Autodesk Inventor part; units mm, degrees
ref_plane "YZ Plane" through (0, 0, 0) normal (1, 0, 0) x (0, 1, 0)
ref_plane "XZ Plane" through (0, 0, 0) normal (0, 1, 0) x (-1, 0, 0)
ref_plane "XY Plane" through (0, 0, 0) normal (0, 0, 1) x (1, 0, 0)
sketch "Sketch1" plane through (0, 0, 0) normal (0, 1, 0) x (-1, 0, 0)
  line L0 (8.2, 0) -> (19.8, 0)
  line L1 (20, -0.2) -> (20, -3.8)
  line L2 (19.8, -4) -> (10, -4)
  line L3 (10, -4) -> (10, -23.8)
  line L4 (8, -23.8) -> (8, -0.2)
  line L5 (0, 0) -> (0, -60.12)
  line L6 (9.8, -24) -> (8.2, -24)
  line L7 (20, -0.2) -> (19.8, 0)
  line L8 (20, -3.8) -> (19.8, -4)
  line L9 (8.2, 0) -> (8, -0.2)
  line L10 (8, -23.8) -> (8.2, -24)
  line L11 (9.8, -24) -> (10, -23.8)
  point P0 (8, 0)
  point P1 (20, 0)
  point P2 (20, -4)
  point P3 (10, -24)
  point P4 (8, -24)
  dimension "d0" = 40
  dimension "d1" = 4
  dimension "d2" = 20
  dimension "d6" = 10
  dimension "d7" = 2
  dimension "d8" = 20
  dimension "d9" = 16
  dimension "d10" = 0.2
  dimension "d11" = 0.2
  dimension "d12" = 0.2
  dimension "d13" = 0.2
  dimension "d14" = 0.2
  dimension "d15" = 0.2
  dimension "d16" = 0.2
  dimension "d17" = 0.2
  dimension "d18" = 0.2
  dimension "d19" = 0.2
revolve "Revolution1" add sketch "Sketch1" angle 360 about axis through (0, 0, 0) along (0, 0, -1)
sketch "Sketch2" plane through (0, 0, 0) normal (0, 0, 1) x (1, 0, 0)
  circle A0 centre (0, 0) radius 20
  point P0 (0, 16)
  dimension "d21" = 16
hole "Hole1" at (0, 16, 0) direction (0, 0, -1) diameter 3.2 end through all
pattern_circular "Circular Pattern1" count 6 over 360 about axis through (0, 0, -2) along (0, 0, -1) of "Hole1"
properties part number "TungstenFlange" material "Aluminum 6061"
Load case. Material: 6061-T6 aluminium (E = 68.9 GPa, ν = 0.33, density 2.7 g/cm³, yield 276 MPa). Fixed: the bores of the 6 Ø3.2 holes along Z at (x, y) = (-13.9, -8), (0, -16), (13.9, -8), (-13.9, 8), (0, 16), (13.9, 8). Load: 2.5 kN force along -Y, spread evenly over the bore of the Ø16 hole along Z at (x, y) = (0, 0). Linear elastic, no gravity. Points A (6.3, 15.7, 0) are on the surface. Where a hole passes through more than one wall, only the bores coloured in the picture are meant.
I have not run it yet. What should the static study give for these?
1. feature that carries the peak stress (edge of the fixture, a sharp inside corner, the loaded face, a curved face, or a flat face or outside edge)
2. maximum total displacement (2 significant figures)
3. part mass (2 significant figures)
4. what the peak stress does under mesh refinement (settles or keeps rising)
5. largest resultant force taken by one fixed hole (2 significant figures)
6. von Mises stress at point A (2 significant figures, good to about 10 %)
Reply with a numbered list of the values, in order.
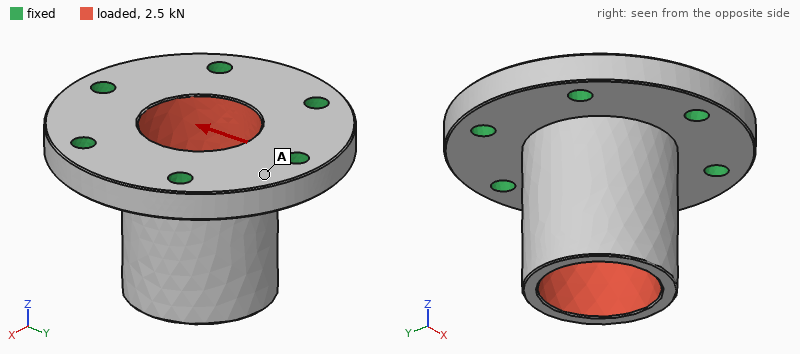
1. edge of the fixture
2. 44 µm
3. 17 g
4. keeps rising
5. 870 N
6. 16 MPa
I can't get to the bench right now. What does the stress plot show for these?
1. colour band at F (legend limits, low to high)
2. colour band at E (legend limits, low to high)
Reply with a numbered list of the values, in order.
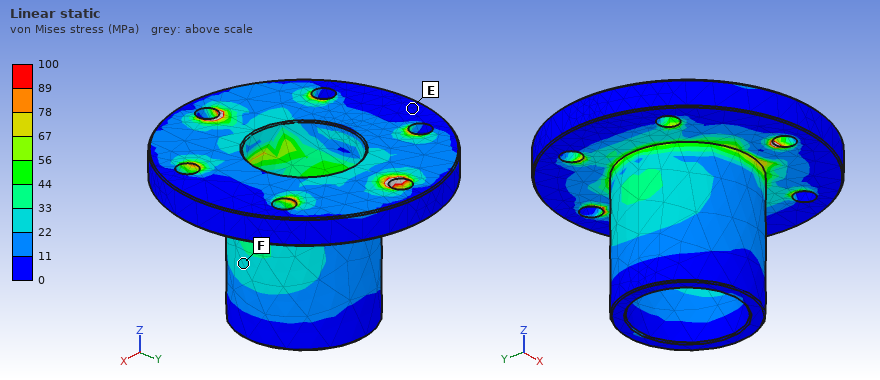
1. 22 to 33 MPa
2. 0 to 11 MPa
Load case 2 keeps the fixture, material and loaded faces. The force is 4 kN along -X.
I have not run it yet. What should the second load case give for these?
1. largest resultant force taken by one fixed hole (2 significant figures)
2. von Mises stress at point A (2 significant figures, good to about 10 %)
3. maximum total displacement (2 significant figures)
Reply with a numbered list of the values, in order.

1. 1.2 kN
2. 16 MPa
3. 71 µm
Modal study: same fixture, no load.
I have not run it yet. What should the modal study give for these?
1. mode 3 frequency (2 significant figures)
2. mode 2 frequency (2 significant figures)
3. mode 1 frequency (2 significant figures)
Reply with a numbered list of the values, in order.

1. 19 kHz
2. 16 kHz
3. 16 kHz
